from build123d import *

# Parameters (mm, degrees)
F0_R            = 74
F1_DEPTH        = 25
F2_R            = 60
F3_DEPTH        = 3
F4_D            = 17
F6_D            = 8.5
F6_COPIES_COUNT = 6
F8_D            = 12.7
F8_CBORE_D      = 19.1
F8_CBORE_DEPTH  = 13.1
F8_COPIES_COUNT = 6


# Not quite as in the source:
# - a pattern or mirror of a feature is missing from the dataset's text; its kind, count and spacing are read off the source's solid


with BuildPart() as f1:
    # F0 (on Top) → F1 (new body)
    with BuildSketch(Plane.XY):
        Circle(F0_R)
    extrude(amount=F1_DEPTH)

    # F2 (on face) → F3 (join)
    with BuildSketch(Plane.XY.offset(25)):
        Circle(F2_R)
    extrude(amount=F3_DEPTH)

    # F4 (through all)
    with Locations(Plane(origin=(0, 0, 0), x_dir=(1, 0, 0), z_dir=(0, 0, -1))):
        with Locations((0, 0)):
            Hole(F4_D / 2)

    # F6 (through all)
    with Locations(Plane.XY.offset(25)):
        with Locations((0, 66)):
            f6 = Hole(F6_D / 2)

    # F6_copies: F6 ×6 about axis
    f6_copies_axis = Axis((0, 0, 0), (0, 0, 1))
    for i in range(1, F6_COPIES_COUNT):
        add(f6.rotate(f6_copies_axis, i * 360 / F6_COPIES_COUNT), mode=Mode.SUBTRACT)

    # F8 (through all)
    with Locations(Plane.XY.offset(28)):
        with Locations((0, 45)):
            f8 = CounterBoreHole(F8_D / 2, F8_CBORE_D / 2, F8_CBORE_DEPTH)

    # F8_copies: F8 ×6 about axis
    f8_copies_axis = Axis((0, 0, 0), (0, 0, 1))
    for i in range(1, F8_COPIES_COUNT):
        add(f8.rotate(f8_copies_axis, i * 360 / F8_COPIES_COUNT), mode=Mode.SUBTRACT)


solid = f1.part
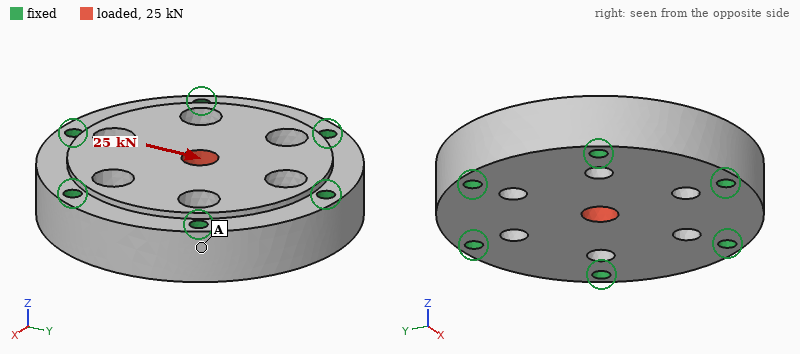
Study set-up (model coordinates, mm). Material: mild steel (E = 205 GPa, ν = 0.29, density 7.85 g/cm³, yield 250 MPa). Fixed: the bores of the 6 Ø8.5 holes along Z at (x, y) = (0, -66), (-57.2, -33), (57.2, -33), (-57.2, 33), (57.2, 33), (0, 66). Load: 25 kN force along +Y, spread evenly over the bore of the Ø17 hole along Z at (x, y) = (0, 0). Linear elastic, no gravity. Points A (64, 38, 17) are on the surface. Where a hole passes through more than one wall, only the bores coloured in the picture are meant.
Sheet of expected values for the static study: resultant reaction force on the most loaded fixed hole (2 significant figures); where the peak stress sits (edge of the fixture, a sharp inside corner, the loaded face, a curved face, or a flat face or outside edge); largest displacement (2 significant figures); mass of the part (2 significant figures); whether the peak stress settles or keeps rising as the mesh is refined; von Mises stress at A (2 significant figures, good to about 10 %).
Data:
6.0 kN
a sharp inside corner
3.7 µm
3.3 kg
keeps rising
4.5 MPa
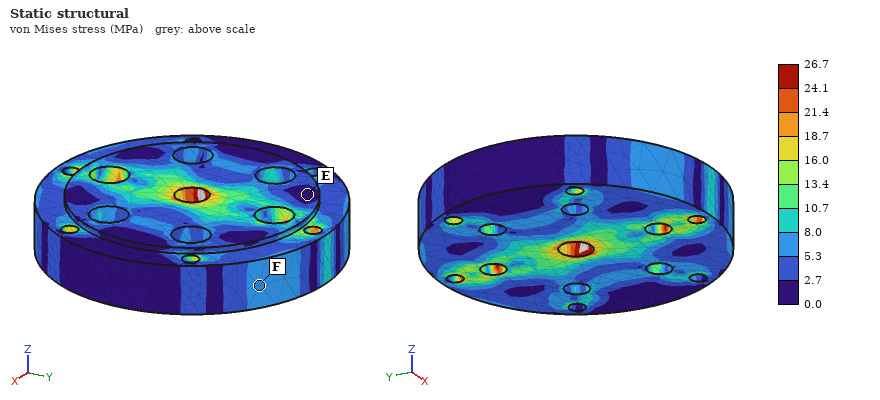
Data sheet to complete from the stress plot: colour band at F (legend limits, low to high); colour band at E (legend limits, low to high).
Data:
5.3 to 8.0 MPa
0.0 to 2.7 MPa
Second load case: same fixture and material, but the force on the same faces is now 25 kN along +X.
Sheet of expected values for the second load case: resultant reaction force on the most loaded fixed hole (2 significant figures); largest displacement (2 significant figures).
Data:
5.3 kN
3.7 µm
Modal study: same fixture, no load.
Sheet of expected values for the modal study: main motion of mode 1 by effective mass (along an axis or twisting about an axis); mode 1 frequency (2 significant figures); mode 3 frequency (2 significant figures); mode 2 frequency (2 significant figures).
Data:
along Z
8200 Hz
14 kHz
14 kHz
